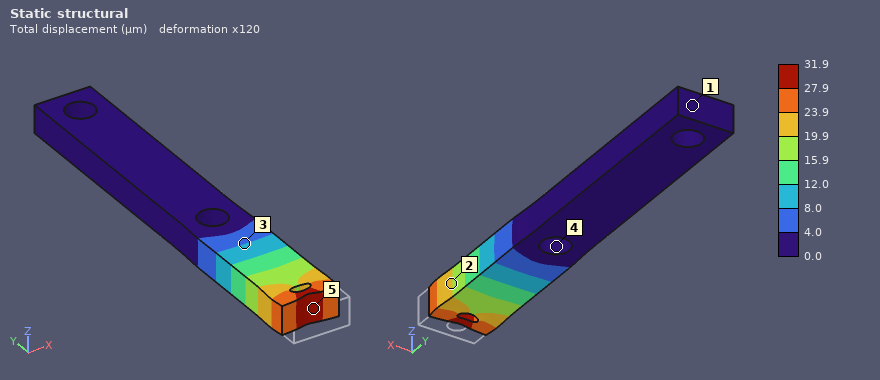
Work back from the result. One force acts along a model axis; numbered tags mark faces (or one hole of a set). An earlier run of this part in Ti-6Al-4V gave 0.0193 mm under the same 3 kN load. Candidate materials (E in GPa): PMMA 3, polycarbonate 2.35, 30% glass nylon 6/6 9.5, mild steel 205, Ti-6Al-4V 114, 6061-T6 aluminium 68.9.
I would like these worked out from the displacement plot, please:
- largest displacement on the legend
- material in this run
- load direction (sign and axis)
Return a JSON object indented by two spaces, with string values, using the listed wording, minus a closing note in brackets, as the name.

{
  "largest displacement on the legend": "31.9 µm",
  "material in this run": "6061-T6 aluminium",
  "load direction": "+Y"
}
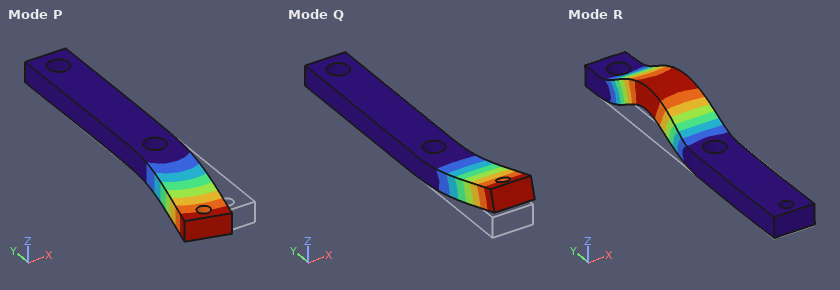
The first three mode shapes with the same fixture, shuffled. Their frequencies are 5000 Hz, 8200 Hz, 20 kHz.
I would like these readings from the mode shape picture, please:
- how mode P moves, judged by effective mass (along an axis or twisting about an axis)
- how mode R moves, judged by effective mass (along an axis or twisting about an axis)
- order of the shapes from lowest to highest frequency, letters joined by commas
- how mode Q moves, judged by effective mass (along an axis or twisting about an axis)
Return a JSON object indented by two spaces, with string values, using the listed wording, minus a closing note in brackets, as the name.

{
  "how mode P moves, judged by effective mass": "along X",
  "how mode R moves, judged by effective mass": "along Z",
  "order of the shapes from lowest to highest frequency, letters joined by commas": "Q, P, R",
  "how mode Q moves, judged by effective mass": "along Z"
}
